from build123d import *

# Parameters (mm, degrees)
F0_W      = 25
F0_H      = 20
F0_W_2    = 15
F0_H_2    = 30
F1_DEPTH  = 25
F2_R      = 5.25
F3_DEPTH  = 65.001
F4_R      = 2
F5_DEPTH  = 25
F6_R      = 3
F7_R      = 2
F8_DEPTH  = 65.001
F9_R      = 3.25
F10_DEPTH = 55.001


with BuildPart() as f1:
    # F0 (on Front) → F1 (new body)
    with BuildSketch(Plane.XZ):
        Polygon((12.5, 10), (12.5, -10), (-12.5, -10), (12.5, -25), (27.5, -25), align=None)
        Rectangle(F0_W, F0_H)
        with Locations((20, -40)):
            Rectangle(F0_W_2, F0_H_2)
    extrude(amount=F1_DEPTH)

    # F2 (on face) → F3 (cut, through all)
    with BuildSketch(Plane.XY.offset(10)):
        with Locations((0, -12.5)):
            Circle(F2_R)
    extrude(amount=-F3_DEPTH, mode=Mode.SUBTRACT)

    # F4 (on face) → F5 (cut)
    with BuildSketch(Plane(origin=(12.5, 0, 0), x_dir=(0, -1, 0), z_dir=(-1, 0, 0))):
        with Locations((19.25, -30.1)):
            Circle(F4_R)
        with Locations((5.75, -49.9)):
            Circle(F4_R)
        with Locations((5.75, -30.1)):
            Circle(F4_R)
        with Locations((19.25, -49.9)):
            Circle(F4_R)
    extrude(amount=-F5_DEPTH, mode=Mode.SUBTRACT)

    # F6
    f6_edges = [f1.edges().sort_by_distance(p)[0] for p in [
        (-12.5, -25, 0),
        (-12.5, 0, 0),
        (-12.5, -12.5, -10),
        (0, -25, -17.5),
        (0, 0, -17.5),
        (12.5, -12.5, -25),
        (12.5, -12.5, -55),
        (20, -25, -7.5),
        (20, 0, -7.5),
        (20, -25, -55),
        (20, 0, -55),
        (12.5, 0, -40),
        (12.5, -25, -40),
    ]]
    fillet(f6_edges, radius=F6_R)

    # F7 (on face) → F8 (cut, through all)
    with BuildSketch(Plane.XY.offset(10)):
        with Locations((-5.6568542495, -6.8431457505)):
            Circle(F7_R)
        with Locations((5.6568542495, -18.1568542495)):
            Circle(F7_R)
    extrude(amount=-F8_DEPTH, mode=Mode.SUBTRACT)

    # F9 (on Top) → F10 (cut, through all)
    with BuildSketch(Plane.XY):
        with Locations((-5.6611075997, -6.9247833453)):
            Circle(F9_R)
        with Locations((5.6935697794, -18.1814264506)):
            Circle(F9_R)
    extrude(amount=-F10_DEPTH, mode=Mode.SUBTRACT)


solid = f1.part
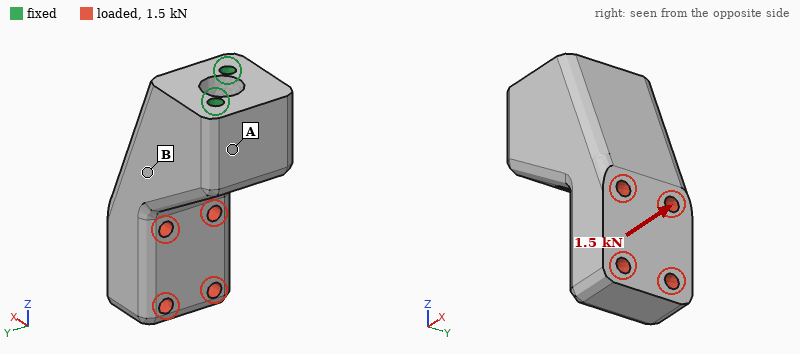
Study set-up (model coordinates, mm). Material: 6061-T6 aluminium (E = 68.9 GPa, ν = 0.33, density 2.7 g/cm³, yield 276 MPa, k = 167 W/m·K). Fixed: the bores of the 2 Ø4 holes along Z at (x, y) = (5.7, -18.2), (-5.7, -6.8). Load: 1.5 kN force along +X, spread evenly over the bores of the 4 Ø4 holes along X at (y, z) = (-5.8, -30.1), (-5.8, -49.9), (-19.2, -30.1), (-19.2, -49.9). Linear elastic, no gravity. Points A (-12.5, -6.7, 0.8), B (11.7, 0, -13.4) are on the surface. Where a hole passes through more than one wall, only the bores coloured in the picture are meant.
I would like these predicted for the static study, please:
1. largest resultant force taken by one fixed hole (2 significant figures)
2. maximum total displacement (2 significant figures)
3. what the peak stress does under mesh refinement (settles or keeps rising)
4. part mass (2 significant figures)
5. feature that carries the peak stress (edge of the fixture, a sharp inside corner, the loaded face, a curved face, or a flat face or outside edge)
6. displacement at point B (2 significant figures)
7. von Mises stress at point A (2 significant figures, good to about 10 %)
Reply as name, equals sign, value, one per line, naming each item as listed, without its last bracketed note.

largest resultant force taken by one fixed hole = 2.2 kN
maximum total displacement = 0.18 mm
what the peak stress does under mesh refinement = keeps rising
part mass = 81 g
feature that carries the peak stress = edge of the fixture
displacement at point B = 0.039 mm
von Mises stress at point A = 41 MPa
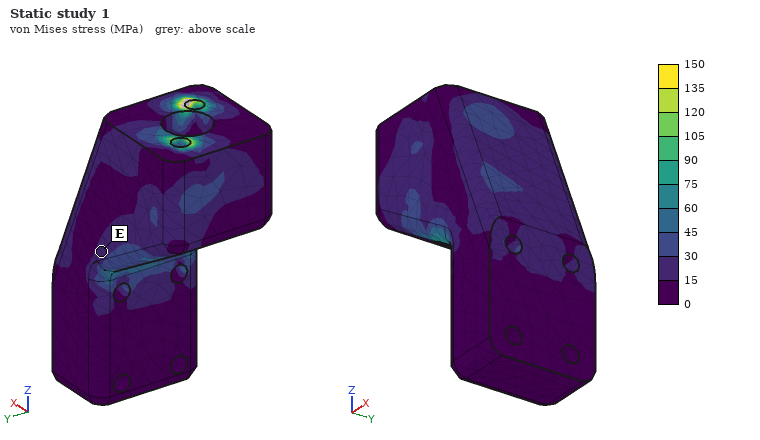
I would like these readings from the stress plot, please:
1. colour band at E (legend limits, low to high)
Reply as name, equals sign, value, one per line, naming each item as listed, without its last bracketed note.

colour band at E = 15 to 30 MPa
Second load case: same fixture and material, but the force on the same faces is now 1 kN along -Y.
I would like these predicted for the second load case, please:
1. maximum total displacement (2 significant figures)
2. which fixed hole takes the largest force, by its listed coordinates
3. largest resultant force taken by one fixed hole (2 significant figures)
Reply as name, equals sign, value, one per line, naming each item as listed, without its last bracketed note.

maximum total displacement = 97 µm
which fixed hole takes the largest force, by its listed coordinates = (5.7, -18.2)
largest resultant force taken by one fixed hole = 1.9 kN
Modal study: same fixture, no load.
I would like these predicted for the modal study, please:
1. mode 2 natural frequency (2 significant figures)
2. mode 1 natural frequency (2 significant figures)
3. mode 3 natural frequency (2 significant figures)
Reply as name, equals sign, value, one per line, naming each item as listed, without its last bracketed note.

mode 2 natural frequency = 4100 Hz
mode 1 natural frequency = 2800 Hz
mode 3 natural frequency = 11 kHz
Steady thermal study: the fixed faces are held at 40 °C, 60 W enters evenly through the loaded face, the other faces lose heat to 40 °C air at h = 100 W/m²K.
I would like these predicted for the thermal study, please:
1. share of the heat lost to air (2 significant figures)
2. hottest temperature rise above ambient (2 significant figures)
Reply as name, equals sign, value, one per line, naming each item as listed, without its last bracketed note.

share of the heat lost to air = 23 %
hottest temperature rise above ambient = 41 K
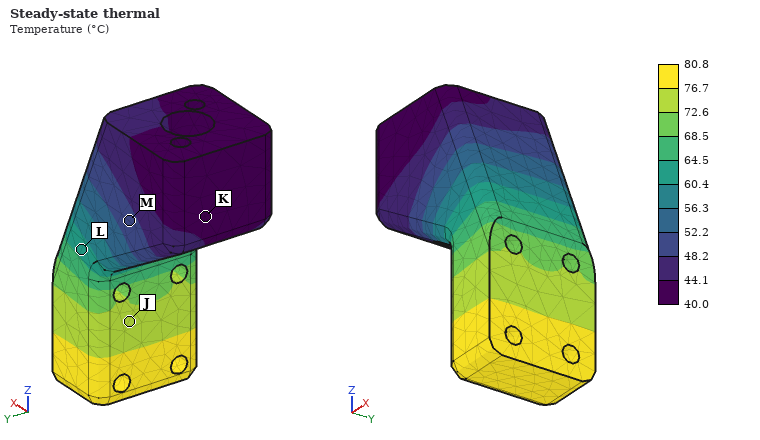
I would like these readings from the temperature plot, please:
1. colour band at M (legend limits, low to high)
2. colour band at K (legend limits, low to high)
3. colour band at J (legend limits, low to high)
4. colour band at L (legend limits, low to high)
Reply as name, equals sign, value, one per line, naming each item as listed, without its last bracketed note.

colour band at M = 48.2 to 52.2 °C
colour band at K = 40.0 to 44.1 °C
colour band at J = 72.6 to 76.7 °C
colour band at L = 60.4 to 64.5 °C
